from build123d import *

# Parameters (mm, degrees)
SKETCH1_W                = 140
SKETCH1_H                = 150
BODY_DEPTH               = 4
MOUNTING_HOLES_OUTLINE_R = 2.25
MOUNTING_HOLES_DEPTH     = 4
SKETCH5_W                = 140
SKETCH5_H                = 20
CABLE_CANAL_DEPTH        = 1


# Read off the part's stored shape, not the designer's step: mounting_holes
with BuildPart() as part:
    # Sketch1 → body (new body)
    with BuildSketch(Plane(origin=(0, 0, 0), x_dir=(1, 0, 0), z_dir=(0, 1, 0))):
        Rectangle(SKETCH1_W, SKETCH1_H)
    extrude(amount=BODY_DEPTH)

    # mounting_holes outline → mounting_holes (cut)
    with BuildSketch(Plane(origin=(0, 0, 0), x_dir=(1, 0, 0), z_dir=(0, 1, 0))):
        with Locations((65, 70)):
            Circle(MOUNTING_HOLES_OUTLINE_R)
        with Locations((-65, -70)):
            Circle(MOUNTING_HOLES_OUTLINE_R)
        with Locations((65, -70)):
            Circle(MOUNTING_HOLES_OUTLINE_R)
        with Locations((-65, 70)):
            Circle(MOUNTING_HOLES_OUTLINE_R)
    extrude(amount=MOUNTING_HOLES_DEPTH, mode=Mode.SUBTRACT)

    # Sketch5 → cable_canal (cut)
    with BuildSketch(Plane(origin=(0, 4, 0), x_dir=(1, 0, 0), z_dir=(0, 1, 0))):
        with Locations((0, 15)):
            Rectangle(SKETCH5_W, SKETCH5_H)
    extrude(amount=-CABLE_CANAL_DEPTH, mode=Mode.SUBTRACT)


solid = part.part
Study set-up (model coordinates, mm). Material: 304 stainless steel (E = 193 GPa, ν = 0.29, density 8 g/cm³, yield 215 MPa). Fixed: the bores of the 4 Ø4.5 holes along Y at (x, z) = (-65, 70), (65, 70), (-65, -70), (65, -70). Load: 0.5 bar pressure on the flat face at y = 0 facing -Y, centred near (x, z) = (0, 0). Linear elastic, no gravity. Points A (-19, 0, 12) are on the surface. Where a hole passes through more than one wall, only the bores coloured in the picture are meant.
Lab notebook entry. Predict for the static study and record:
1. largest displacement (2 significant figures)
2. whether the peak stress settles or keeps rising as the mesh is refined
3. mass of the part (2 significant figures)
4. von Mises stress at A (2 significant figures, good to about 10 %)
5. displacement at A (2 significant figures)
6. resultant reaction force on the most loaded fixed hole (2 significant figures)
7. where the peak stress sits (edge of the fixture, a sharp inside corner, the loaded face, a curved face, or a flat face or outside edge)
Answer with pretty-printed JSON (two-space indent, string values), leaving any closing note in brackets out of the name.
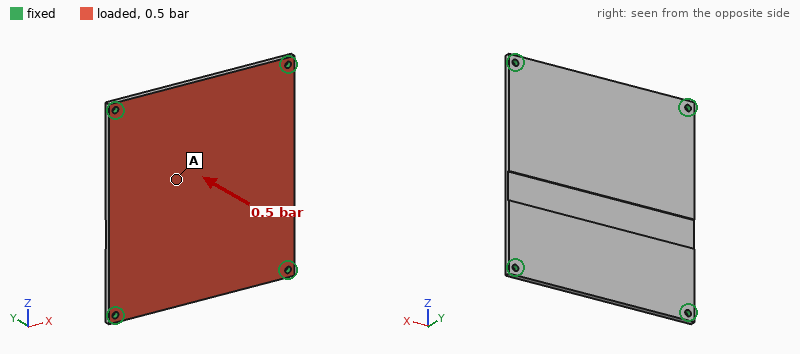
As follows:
{
  "largest displacement": "0.17 mm",
  "whether the peak stress settles or keeps rising as the mesh is refined": "keeps rising",
  "mass of the part": "650 g",
  "von Mises stress at A": "19 MPa",
  "displacement at A": "0.15 mm",
  "resultant reaction force on the most loaded fixed hole": "320 N",
  "where the peak stress sits": "edge of the fixture"
}
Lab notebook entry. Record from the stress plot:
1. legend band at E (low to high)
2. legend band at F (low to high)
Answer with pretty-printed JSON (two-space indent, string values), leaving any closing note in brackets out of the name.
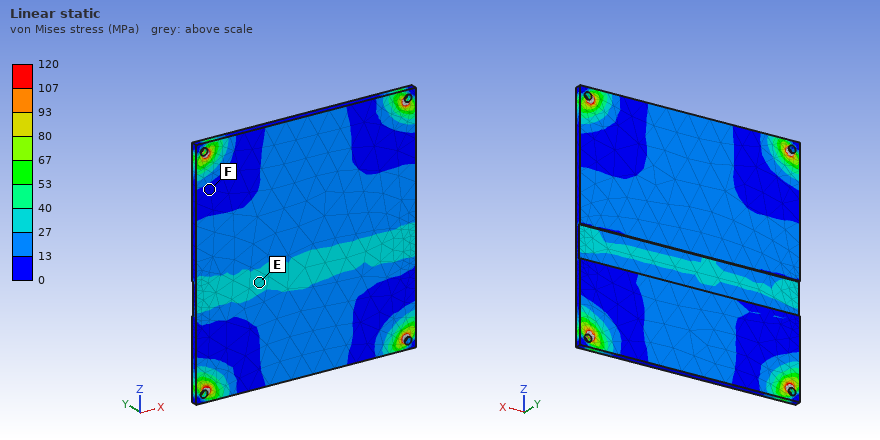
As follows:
{
  "legend band at E": "27 to 40 MPa",
  "legend band at F": "0 to 13 MPa"
}
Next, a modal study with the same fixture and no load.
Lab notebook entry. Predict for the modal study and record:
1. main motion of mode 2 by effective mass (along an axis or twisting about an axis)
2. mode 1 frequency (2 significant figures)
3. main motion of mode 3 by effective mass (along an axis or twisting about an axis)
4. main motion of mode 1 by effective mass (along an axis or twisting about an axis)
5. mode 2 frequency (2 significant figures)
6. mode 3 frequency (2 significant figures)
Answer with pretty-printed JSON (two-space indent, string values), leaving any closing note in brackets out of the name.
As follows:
{
  "main motion of mode 2 by effective mass": "twisting about Z",
  "mode 1 frequency": "610 Hz",
  "main motion of mode 3 by effective mass": "twisting about X",
  "main motion of mode 1 by effective mass": "along Y",
  "mode 2 frequency": "1100 Hz",
  "mode 3 frequency": "1200 Hz"
}
